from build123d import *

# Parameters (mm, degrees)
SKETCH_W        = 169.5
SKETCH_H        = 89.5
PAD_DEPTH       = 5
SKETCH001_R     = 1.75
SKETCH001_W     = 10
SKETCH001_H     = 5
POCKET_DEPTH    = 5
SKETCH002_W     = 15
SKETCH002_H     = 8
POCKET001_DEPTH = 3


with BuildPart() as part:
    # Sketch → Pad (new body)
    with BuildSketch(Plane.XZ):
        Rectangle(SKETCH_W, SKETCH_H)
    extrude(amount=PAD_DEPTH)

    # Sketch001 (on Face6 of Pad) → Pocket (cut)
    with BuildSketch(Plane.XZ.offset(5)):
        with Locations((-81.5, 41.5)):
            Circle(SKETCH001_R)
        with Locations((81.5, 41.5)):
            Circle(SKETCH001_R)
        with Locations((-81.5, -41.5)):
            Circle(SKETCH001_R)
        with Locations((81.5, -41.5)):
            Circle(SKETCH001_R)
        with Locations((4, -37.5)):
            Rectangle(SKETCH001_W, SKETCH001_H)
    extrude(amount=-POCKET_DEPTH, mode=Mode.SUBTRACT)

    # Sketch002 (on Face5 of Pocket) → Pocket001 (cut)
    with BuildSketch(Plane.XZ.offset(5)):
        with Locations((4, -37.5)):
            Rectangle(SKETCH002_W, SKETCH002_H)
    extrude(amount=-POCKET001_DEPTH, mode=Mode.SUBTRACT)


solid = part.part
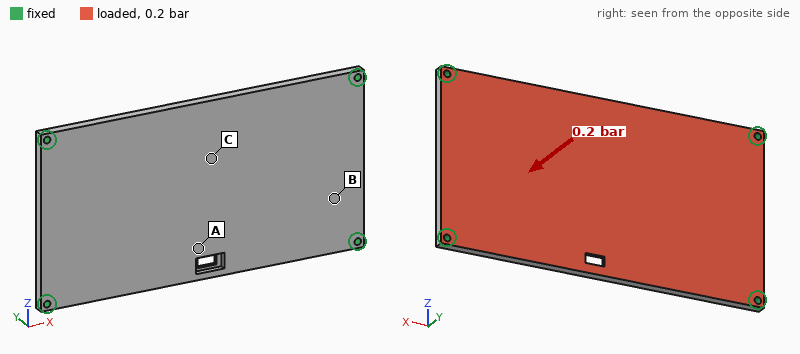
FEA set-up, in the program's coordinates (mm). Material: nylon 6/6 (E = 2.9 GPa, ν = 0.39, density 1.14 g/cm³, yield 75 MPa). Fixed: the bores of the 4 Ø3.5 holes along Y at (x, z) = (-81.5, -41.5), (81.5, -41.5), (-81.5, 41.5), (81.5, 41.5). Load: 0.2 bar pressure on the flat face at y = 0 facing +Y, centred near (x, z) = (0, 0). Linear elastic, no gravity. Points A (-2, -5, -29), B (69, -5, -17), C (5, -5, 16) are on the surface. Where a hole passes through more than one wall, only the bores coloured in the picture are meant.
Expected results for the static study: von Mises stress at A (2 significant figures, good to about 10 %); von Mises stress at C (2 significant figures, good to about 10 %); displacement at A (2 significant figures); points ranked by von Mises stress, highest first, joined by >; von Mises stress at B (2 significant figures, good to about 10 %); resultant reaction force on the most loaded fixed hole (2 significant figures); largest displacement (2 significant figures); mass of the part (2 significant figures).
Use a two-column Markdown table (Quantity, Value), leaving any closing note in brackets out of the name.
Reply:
| Quantity | Value |
|---|---|
| von Mises stress at A | 8.4 MPa |
| von Mises stress at C | 6.7 MPa |
| displacement at A | 2.2 mm |
| points ranked by von Mises stress, highest first, joined by > | A > C > B |
| von Mises stress at B | 2.7 MPa |
| resultant reaction force on the most loaded fixed hole | 76 N |
| largest displacement | 2.3 mm |
| mass of the part | 86 g |
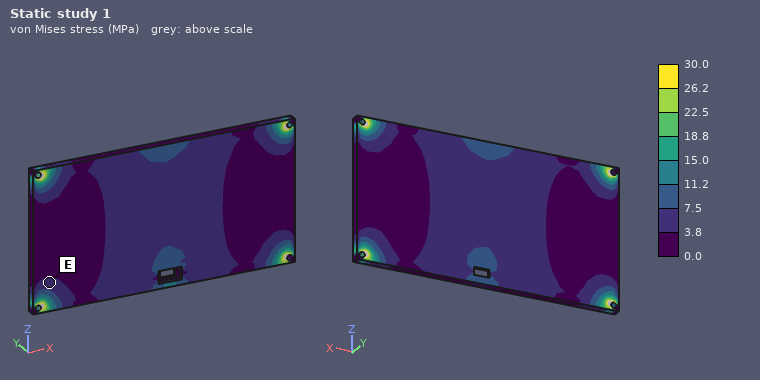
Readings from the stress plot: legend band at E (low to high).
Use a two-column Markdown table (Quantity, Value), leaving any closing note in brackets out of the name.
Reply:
| Quantity | Value |
|---|---|
| legend band at E | 3.8 to 7.5 MPa |
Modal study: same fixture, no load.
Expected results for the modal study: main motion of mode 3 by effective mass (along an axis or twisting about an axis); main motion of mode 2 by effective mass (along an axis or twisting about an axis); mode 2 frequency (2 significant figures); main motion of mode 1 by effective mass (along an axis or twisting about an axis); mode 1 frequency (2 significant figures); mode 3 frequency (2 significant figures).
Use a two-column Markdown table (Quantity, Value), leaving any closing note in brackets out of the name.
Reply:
| Quantity | Value |
|---|---|
| main motion of mode 3 by effective mass | twisting about Z |
| main motion of mode 2 by effective mass | twisting about X |
| mode 2 frequency | 460 Hz |
| main motion of mode 1 by effective mass | along Y |
| mode 1 frequency | 230 Hz |
| mode 3 frequency | 670 Hz |
